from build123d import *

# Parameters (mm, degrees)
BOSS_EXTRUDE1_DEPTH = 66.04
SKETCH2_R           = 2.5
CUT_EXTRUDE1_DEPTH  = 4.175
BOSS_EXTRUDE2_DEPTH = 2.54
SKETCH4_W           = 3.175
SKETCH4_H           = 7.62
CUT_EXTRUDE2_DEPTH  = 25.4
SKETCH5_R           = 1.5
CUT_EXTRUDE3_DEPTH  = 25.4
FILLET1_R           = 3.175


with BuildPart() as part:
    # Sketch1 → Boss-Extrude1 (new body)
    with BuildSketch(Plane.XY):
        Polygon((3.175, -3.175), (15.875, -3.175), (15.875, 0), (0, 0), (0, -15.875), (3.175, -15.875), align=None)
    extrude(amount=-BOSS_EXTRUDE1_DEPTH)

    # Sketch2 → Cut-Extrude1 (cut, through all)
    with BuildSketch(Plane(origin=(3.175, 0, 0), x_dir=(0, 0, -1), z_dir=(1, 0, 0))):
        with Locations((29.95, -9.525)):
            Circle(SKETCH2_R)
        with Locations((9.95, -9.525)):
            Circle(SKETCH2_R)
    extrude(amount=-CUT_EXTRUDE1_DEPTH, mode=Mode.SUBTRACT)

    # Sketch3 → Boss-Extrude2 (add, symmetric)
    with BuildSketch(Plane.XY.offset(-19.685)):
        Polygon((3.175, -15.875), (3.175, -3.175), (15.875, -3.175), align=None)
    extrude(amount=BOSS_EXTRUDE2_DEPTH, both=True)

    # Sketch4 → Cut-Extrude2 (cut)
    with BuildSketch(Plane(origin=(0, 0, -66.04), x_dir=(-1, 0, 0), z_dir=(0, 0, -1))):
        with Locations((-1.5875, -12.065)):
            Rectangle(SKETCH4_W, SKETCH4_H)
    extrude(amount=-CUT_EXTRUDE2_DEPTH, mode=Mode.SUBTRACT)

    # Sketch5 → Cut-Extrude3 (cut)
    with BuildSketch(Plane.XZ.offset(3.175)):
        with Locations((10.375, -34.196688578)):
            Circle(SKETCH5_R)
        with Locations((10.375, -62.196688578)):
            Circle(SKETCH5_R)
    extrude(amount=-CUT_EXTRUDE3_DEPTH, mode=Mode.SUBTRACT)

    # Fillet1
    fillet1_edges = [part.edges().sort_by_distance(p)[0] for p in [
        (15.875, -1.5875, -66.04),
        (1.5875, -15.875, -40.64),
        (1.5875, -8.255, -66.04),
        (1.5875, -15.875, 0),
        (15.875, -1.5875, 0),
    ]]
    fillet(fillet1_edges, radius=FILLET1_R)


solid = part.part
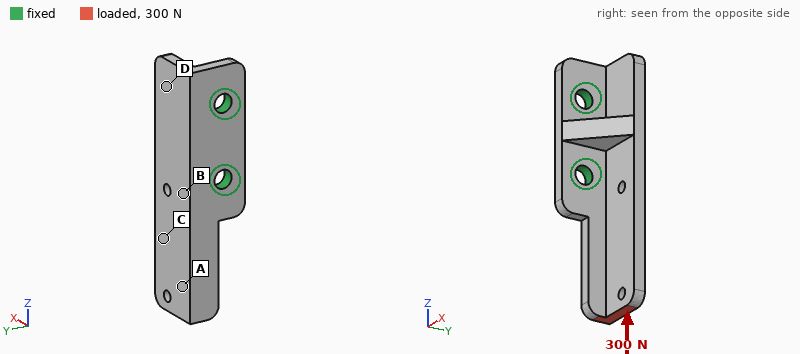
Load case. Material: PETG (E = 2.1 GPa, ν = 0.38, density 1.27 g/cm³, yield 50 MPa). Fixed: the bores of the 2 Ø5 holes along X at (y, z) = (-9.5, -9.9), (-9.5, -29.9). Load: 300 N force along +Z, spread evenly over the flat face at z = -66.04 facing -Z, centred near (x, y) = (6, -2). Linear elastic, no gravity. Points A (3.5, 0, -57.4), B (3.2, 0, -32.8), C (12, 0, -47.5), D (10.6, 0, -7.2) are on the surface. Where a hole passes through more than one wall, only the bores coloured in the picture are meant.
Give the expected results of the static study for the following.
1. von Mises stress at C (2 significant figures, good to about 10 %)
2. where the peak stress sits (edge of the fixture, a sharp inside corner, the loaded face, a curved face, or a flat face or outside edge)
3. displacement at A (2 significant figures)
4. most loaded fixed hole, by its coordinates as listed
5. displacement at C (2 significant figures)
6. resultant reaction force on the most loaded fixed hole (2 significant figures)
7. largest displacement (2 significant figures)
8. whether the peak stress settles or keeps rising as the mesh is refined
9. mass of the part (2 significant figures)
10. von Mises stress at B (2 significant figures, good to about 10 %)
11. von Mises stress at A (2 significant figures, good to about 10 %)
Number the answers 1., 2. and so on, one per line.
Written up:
1. 5.5 MPa
2. edge of the fixture
3. 0.32 mm
4. (-9.5, -29.9)
5. 0.18 mm
6. 210 N
7. 0.49 mm
8. keeps rising
9. 7.1 g
10. 7.4 MPa
11. 8.6 MPa
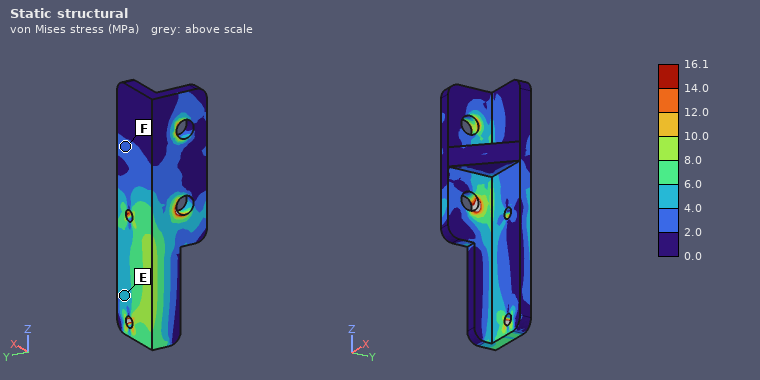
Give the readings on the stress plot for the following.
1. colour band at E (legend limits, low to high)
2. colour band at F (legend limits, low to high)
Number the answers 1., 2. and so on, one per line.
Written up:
1. 4.0 to 6.0 MPa
2. 2.0 to 4.0 MPa
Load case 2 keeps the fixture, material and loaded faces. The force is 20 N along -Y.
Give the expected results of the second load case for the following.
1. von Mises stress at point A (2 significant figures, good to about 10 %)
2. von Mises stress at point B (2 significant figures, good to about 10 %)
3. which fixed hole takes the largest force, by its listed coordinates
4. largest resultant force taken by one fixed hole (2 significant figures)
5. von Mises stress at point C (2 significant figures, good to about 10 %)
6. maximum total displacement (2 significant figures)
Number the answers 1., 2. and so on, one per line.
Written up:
1. 2.9 MPa
2. 4.5 MPa
3. (-9.5, -29.9)
4. 46 N
5. 2.9 MPa
6. 0.71 mm
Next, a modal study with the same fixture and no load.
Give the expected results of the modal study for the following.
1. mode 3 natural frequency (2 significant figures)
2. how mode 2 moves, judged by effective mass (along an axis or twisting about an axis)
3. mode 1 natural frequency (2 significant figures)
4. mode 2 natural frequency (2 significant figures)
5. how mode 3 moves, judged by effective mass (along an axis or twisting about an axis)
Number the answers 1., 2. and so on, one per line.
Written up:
1. 2000 Hz
2. along X
3. 970 Hz
4. 1500 Hz
5. twisting about Z
